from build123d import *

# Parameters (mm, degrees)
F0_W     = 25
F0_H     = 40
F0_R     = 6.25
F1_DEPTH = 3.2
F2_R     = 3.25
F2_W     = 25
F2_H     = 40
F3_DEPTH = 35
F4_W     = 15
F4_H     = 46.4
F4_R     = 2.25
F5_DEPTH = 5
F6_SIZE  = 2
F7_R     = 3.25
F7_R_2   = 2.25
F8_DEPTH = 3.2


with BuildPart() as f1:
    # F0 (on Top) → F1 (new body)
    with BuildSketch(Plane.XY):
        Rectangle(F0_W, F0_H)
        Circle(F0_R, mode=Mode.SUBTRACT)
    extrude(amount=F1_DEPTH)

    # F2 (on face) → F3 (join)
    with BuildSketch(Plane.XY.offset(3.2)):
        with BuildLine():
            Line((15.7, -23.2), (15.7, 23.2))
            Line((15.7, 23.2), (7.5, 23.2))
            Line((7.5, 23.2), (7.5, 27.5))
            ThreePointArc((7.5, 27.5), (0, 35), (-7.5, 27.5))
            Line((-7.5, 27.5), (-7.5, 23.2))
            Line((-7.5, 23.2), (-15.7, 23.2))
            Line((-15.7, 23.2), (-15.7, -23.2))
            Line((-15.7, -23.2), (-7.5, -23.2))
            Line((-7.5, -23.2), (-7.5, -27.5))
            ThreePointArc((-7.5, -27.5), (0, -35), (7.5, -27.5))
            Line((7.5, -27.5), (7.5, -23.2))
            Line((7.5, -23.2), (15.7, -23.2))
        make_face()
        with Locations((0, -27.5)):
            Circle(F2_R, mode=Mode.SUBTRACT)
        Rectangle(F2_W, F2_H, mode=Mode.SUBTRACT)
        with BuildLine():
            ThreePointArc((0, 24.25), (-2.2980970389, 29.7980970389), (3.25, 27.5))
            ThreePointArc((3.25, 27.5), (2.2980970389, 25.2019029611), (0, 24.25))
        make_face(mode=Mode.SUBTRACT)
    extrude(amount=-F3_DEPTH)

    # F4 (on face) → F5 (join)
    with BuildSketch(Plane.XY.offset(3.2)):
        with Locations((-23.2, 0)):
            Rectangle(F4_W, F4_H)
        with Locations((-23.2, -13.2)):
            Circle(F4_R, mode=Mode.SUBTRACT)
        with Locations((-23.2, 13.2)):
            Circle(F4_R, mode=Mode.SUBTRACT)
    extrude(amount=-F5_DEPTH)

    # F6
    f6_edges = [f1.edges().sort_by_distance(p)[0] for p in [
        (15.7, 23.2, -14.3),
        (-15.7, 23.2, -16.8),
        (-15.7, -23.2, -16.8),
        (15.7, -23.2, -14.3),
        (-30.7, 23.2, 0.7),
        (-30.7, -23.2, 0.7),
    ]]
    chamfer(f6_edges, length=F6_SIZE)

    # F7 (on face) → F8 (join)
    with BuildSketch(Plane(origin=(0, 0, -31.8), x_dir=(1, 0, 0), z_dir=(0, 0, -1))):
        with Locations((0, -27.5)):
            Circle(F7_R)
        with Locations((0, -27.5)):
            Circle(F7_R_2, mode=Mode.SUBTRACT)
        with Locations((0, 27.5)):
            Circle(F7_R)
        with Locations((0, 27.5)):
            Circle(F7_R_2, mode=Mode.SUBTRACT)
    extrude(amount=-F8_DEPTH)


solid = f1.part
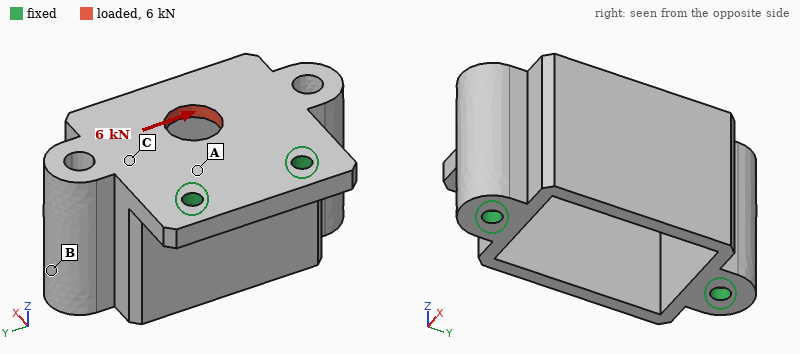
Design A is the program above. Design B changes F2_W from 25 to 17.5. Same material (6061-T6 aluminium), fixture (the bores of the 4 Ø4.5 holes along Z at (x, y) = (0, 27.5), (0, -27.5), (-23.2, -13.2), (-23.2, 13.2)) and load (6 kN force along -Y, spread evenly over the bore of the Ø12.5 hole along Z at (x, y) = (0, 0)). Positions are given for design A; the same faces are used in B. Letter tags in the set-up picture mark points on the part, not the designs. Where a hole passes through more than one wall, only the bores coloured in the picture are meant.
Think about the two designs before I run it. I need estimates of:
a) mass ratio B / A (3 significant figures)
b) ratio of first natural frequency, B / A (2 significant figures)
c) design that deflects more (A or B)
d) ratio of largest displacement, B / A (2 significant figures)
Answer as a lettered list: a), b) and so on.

a) 1.31
b) 1.2
c) A
d) 0.64
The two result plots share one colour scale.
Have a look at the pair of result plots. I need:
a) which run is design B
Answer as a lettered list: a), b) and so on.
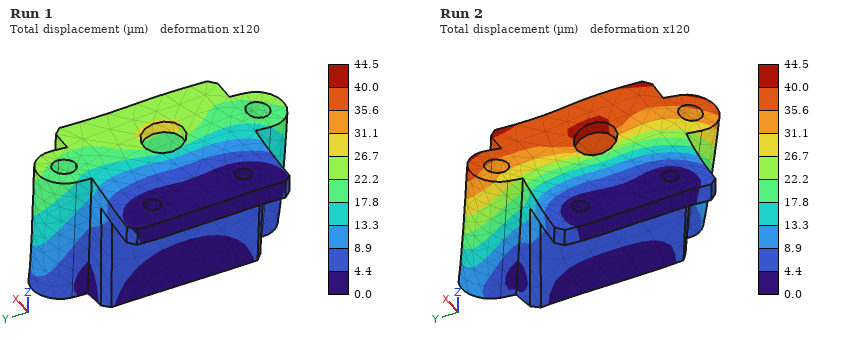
a) Run 1
